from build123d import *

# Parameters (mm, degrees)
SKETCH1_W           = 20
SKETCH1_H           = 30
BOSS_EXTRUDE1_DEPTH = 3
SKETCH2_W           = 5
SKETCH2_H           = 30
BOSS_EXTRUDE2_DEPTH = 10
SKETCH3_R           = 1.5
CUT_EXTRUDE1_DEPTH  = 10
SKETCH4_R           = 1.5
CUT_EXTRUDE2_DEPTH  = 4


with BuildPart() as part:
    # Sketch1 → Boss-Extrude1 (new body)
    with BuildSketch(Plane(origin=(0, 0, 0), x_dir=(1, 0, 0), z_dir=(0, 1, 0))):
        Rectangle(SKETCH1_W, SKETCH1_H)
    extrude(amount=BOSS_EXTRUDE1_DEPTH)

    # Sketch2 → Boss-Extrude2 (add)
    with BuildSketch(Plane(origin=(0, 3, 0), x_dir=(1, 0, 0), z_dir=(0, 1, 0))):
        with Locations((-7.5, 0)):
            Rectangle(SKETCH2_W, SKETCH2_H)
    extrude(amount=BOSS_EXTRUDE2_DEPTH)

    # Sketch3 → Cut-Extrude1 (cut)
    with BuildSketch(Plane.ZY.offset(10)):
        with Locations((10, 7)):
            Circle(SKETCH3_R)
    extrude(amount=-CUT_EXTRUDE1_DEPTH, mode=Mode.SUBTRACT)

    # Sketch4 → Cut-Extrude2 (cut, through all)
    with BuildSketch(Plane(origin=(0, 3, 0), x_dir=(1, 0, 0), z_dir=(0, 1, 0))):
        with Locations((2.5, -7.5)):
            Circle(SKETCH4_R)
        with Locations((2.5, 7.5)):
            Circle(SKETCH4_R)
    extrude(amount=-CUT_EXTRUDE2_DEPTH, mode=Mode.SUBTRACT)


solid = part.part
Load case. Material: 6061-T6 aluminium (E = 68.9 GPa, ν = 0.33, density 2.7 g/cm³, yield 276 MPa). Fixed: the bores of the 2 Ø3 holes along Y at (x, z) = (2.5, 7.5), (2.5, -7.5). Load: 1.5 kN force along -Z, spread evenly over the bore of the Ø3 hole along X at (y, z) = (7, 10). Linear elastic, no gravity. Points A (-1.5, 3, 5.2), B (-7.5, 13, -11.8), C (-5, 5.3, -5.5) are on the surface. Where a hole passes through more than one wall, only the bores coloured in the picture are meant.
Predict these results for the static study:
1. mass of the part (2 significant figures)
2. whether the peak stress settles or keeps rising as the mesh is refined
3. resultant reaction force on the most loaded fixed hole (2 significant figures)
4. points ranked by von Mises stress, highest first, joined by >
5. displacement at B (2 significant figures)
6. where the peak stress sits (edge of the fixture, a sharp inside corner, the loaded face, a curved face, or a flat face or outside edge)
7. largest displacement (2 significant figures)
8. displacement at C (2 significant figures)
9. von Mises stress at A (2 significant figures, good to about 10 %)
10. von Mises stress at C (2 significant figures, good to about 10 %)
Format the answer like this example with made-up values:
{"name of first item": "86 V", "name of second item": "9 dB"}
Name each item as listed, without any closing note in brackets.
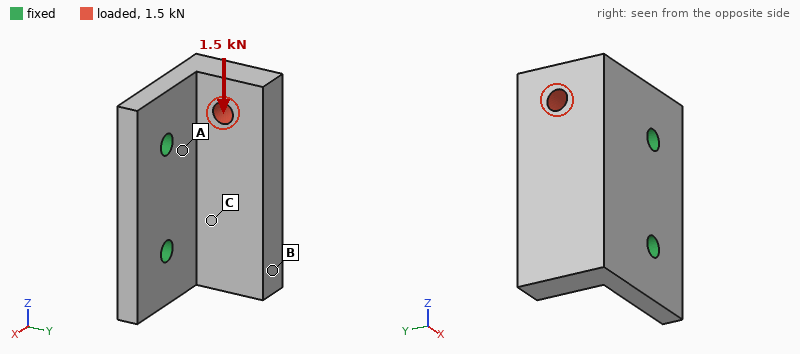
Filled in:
{"mass of the part": "8.7 g", "whether the peak stress settles or keeps rising as the mesh is refined": "keeps rising", "resultant reaction force on the most loaded fixed hole": "1.2 kN", "points ranked by von Mises stress, highest first, joined by >": "A > C > B", "displacement at B": "50 µm", "where the peak stress sits": "edge of the fixture", "largest displacement": "59 µm", "displacement at C": "23 µm", "von Mises stress at A": "88 MPa", "von Mises stress at C": "43 MPa"}
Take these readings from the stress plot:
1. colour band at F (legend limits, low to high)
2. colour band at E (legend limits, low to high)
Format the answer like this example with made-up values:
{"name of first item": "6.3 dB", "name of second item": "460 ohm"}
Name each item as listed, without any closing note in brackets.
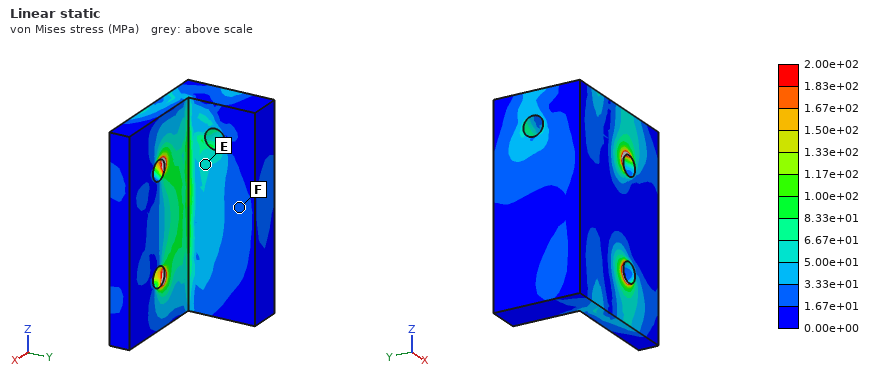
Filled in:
{"colour band at F": "1.67e+01 to 3.33e+01 MPa", "colour band at E": "5.00e+01 to 6.67e+01 MPa"}
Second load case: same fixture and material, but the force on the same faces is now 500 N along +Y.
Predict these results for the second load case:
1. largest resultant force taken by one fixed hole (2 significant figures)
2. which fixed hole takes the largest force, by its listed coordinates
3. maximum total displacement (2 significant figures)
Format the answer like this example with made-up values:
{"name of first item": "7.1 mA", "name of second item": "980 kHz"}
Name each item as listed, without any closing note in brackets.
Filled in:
{"largest resultant force taken by one fixed hole": "520 N", "which fixed hole takes the largest force, by its listed coordinates": "(2.5, 7.5)", "maximum total displacement": "0.11 mm"}
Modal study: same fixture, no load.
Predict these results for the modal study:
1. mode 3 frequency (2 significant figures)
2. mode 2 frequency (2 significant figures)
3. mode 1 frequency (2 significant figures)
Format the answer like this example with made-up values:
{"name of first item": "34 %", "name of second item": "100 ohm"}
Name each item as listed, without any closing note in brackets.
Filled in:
{"mode 3 frequency": "20 kHz", "mode 2 frequency": "11 kHz", "mode 1 frequency": "5800 Hz"}
